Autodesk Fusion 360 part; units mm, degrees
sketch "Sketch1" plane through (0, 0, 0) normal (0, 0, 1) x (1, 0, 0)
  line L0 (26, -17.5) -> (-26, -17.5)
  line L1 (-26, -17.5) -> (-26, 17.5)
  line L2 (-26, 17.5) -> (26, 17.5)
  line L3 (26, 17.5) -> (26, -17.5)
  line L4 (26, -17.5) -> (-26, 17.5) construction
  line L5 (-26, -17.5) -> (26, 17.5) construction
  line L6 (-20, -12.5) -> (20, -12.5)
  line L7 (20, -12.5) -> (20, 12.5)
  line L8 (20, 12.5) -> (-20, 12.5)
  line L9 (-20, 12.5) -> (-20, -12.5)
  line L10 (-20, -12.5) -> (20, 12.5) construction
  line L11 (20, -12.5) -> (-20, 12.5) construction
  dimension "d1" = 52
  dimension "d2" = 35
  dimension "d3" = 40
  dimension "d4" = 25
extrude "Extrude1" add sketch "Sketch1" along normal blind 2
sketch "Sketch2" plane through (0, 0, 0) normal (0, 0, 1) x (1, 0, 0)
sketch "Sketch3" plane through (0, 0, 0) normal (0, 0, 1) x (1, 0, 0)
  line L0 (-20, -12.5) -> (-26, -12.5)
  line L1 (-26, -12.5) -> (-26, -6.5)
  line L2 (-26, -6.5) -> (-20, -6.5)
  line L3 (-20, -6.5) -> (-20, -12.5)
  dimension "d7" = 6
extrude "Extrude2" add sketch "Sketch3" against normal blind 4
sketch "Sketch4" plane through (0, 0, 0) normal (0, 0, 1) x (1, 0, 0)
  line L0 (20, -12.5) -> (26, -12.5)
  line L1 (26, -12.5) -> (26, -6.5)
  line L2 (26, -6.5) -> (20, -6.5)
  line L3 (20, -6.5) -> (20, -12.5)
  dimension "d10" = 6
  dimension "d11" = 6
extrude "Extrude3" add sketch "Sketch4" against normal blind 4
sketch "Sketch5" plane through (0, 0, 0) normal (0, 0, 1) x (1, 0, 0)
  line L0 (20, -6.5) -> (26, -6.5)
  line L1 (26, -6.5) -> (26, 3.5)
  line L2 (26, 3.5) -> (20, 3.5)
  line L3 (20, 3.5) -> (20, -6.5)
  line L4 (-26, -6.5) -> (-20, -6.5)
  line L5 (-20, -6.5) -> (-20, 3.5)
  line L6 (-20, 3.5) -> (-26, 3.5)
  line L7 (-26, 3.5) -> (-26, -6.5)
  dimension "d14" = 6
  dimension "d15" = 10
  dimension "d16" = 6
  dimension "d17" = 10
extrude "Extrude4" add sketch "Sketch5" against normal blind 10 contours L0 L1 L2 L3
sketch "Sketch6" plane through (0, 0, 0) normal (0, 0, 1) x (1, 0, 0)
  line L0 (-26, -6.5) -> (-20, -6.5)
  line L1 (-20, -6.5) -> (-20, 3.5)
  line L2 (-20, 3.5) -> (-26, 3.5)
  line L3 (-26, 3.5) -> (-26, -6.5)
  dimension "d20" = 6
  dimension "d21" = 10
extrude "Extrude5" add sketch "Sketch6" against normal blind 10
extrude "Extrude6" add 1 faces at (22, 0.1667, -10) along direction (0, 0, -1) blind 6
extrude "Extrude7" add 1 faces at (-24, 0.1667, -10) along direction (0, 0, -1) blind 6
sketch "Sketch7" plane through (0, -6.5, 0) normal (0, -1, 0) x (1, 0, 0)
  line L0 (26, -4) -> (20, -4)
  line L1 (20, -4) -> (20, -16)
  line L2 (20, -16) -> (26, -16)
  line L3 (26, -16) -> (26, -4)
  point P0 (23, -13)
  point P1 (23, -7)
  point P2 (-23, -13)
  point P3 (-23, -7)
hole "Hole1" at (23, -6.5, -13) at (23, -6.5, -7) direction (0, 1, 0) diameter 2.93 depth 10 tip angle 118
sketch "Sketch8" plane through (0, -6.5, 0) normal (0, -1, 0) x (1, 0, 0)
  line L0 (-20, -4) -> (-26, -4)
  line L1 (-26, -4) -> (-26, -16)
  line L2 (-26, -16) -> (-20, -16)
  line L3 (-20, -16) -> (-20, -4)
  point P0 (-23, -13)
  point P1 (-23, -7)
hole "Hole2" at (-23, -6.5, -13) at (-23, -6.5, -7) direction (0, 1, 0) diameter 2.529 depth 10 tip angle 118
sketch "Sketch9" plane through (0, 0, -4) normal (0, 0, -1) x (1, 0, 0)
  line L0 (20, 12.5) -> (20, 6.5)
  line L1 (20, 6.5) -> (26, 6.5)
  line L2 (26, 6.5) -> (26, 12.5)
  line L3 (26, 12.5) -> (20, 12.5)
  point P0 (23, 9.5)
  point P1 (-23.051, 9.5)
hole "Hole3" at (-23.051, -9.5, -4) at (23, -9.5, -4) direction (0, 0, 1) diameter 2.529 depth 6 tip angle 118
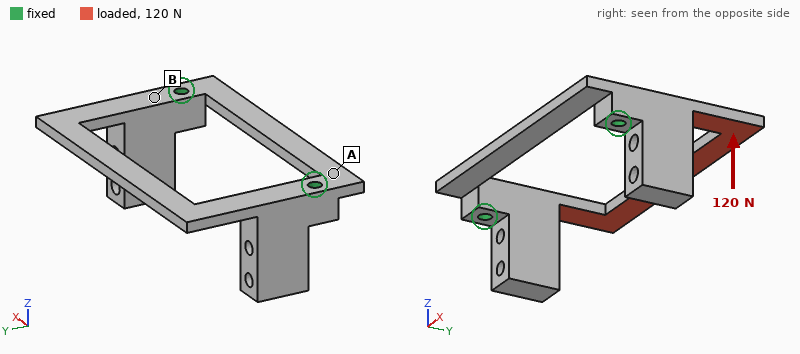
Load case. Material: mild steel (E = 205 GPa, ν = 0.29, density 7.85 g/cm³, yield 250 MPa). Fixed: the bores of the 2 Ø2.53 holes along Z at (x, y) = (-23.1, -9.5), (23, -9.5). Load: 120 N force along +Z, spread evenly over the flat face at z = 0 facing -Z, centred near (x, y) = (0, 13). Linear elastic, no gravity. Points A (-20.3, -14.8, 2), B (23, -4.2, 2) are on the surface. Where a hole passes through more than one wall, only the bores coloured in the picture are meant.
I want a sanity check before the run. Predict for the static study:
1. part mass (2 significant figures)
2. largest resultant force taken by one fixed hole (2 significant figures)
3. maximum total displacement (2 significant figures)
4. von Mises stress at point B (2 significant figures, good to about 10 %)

28 g
60 N
0.11 mm
23 MPa
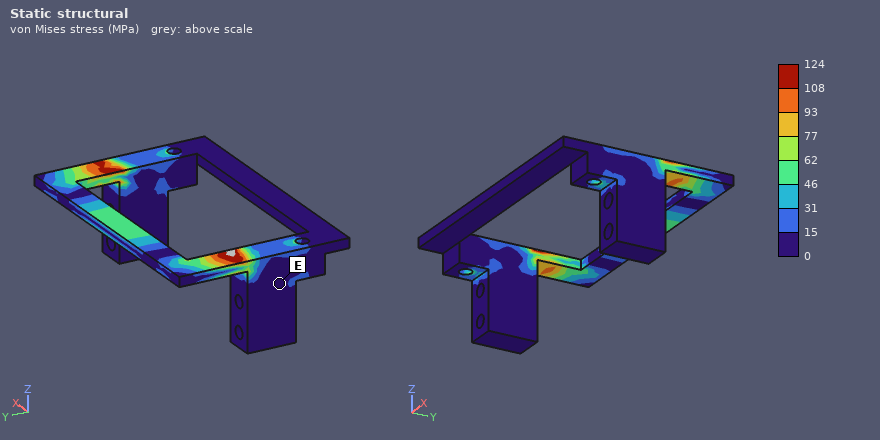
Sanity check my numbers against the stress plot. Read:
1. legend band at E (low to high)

0 to 15 MPa
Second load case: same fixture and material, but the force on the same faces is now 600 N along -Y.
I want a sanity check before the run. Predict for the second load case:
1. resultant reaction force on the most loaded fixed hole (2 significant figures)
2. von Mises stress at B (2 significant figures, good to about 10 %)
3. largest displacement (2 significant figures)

320 N
21 MPa
51 µm
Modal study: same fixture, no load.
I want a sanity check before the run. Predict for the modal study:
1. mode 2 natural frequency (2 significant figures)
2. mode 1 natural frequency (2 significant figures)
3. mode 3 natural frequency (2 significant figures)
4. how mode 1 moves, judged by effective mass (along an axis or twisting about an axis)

5000 Hz
2700 Hz
5400 Hz
along Z
